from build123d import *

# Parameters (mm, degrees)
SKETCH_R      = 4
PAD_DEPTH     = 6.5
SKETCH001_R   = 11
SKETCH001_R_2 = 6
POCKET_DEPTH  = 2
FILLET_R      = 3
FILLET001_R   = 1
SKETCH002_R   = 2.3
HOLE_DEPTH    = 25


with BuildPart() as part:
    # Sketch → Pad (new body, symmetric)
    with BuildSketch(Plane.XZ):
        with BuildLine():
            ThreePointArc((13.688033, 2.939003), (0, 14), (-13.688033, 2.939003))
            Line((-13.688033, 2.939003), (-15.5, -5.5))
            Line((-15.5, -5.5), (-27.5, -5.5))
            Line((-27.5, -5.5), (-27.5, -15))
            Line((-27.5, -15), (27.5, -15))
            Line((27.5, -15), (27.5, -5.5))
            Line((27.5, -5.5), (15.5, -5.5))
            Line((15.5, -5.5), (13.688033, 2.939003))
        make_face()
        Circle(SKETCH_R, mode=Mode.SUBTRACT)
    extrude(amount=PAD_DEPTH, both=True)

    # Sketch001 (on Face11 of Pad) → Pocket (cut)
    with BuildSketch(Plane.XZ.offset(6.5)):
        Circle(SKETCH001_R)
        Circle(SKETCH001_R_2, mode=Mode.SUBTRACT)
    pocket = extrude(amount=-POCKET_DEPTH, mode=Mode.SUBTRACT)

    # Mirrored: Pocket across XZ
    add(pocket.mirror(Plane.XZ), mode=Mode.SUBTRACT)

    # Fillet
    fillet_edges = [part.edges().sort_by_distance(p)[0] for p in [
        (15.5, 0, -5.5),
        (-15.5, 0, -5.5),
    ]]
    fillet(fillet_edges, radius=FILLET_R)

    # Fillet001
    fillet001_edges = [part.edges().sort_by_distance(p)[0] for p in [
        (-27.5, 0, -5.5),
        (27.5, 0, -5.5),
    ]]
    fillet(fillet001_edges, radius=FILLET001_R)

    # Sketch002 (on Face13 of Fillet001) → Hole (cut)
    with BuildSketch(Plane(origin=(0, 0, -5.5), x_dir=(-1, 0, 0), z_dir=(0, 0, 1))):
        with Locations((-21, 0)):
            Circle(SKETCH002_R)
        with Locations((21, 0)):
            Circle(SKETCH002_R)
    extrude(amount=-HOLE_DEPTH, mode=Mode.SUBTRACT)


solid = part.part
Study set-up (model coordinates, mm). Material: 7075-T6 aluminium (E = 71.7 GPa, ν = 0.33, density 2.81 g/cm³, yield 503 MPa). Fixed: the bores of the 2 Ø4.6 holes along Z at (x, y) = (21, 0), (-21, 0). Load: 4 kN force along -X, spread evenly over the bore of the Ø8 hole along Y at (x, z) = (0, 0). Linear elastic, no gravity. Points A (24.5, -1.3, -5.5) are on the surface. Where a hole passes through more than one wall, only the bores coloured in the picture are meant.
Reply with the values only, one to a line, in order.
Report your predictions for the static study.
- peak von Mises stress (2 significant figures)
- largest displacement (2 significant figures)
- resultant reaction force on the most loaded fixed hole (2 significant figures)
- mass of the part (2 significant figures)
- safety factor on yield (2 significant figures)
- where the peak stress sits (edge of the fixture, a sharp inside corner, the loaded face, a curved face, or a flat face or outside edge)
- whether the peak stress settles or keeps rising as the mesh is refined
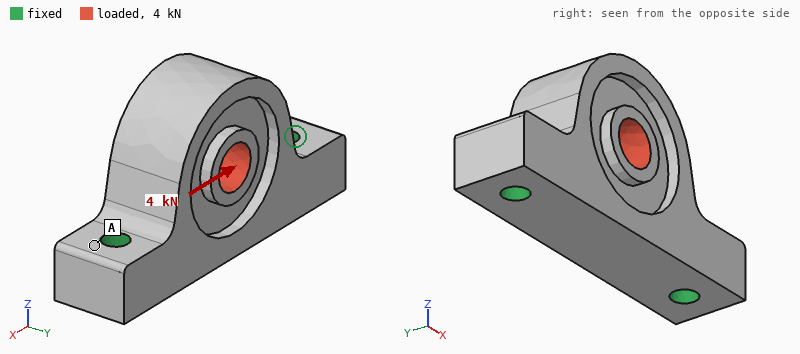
79 MPa
12 µm
2.3 kN
31 g
6.3
a curved face
settles
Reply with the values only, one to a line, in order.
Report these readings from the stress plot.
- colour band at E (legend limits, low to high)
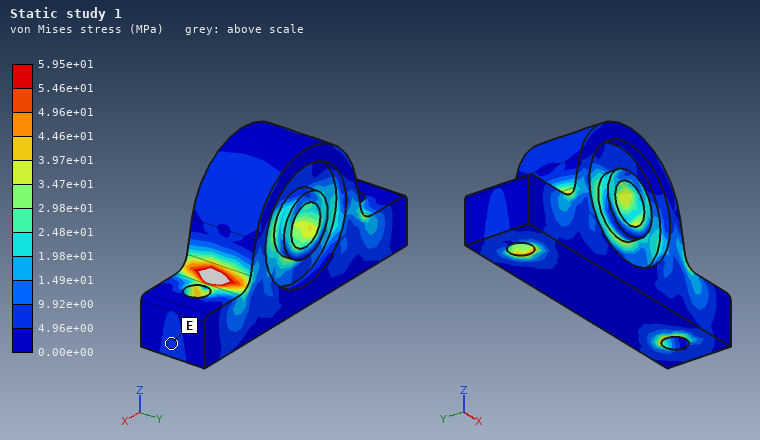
4.96e+00 to 9.92e+00 MPa
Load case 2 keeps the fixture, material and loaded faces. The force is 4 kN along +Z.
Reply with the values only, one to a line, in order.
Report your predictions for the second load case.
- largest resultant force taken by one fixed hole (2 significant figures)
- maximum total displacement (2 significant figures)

2.2 kN
15 µm
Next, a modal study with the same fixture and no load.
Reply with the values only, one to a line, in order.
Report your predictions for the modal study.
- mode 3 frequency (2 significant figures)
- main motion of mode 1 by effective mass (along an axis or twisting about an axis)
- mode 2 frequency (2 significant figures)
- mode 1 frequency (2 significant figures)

23 kHz
along Y
22 kHz
9200 Hz
